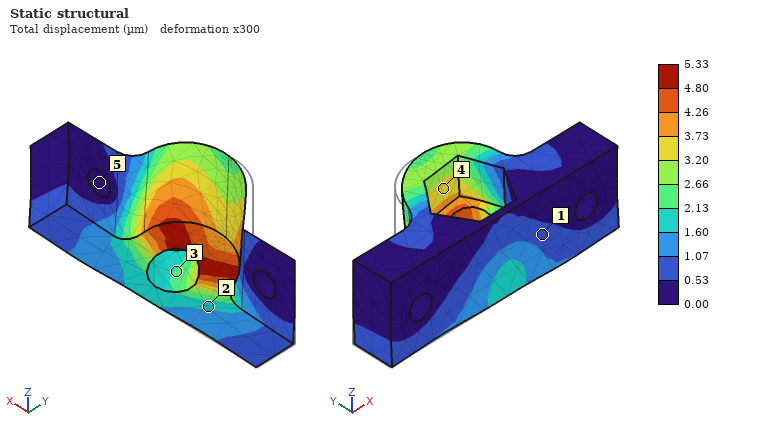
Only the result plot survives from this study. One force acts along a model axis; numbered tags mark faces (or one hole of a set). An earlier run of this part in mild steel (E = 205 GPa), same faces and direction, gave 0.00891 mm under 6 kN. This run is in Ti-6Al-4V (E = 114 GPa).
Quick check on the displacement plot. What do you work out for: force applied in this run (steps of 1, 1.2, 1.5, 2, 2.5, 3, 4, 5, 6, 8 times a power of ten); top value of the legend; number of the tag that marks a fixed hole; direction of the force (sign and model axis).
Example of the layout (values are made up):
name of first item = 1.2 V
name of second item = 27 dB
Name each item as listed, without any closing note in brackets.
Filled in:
force applied in this run = 2 kN
top value of the legend = 5.33 µm
number of the tag that marks a fixed hole = 5
direction of the force = +X
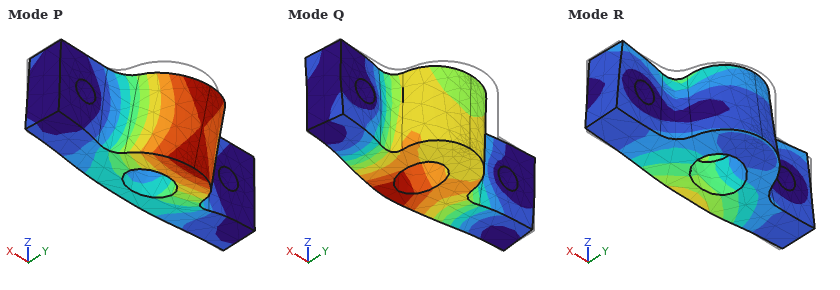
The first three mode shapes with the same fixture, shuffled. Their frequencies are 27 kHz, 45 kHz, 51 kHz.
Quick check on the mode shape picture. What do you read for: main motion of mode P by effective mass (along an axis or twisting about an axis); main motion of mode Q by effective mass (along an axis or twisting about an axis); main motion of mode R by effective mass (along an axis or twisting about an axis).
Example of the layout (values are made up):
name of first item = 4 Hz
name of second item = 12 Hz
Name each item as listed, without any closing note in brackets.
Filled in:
main motion of mode P by effective mass = along Z
main motion of mode Q by effective mass = along Y
main motion of mode R by effective mass = along Z
